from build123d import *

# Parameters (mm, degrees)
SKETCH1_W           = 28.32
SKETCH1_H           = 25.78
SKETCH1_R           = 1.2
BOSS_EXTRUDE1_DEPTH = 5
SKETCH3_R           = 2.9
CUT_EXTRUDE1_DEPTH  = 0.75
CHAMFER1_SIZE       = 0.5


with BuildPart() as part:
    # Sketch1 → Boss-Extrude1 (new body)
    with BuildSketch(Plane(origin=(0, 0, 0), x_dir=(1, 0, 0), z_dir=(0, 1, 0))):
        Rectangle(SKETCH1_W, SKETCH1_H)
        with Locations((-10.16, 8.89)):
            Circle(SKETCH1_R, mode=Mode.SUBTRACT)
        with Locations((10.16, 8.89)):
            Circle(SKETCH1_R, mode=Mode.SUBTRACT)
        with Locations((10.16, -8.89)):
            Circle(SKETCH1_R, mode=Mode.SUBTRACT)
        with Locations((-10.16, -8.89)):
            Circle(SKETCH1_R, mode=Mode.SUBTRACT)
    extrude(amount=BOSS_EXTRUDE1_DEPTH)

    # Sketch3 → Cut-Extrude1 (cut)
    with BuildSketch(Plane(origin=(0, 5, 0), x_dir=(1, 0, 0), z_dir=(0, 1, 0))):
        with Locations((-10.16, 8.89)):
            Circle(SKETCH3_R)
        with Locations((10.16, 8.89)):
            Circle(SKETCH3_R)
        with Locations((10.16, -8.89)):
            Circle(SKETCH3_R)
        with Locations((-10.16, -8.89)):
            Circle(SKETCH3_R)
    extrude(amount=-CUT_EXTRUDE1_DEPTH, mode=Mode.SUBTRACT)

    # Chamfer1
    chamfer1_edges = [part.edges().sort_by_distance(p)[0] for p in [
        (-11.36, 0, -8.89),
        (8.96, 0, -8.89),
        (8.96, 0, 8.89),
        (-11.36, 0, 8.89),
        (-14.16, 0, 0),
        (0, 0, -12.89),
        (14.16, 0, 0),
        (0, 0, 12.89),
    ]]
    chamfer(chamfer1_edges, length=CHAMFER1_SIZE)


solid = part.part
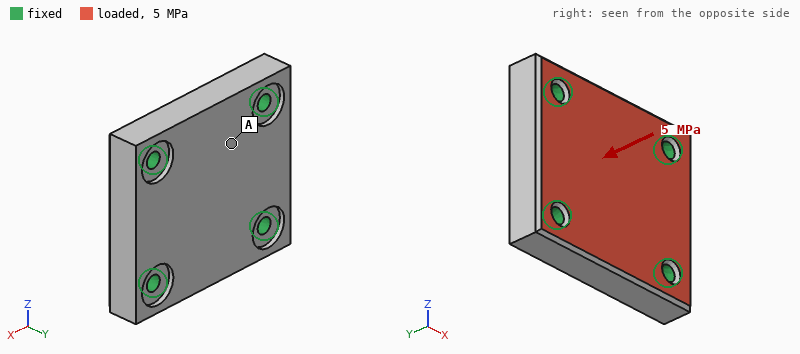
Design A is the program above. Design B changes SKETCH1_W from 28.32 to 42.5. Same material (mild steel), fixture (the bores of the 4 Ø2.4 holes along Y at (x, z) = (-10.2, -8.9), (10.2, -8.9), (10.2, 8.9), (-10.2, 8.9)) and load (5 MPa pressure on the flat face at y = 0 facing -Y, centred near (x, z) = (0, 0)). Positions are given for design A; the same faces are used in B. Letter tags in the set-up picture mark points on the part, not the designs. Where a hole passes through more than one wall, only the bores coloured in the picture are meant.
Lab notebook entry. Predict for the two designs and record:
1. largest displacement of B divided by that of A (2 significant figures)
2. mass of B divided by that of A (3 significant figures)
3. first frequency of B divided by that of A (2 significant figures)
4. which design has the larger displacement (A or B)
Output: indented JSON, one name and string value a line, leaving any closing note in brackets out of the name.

{
  "largest displacement of B divided by that of A": "2.4",
  "mass of B divided by that of A": "1.52",
  "first frequency of B divided by that of A": "0.61",
  "which design has the larger displacement": "B"
}
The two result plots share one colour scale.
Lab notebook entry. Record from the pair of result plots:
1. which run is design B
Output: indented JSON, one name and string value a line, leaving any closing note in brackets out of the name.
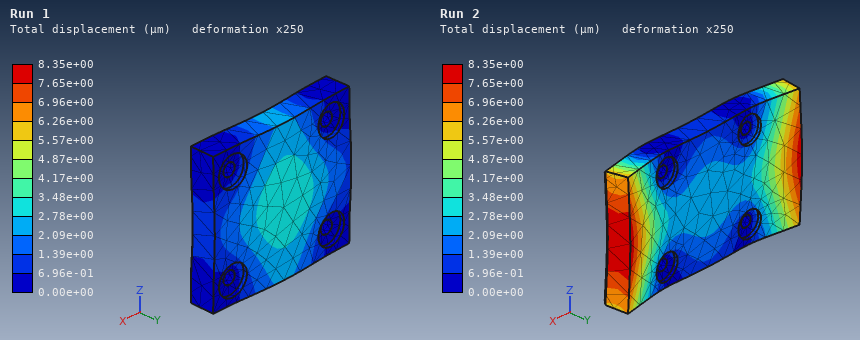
{
  "which run is design B": "Run 2"
}
